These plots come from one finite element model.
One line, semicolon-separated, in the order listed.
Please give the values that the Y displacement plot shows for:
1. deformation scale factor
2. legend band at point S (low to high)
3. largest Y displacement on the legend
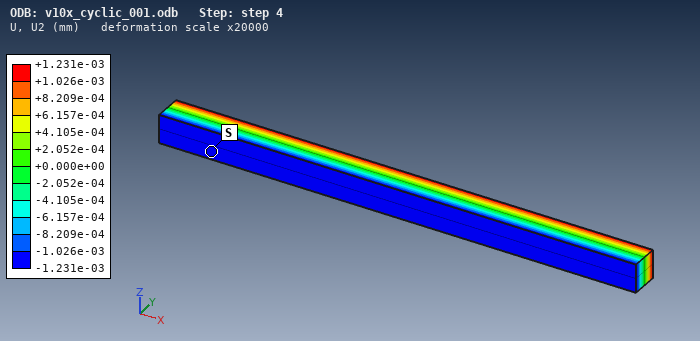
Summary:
20000; -1.231e-03 to -1.026e-03 mm; +1.231e-03 mm
